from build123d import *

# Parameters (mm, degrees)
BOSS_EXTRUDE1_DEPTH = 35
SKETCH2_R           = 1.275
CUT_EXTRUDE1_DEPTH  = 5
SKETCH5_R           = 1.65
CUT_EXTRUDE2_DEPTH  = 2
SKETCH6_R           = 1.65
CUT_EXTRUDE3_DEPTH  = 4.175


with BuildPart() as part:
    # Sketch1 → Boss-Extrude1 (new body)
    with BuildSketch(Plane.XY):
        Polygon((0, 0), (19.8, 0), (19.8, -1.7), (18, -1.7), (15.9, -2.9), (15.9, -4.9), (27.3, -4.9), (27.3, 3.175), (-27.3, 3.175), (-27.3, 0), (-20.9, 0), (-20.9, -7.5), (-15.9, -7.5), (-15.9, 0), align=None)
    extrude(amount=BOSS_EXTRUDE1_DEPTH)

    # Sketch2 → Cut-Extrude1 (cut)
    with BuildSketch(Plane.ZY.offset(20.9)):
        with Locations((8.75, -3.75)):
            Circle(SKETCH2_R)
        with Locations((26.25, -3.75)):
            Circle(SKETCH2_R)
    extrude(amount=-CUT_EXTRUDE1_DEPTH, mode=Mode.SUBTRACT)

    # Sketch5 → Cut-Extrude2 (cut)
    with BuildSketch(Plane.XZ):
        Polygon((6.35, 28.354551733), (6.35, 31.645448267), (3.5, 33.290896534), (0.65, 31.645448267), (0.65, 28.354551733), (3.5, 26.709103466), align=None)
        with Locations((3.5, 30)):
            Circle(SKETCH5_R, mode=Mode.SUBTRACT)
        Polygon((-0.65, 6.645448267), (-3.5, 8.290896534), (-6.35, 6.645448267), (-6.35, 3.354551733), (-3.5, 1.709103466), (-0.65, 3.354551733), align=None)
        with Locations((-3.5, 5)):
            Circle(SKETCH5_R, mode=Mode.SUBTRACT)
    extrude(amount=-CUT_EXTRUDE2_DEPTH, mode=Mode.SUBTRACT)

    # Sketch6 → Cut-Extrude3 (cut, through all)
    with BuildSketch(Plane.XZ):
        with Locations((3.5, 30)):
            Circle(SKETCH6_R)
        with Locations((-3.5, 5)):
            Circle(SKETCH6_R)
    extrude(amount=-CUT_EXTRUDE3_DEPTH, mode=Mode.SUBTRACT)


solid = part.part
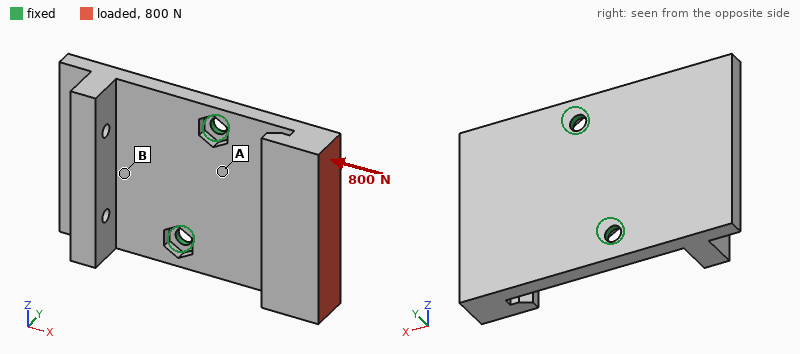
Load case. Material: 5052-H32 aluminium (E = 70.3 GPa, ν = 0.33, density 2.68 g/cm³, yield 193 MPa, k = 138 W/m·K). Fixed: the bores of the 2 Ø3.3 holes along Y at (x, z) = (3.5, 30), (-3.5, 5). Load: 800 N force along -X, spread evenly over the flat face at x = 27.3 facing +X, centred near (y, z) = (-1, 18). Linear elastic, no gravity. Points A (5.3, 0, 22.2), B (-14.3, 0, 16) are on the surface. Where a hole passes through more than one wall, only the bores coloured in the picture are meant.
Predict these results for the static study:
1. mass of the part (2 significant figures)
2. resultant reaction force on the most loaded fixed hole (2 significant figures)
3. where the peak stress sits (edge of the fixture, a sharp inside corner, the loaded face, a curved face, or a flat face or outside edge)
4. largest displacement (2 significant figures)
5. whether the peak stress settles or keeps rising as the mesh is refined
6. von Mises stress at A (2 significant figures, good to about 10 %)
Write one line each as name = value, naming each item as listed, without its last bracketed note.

mass of the part = 24 g
resultant reaction force on the most loaded fixed hole = 400 N
where the peak stress sits = edge of the fixture
largest displacement = 0.25 mm
whether the peak stress settles or keeps rising as the mesh is refined = keeps rising
von Mises stress at A = 43 MPa
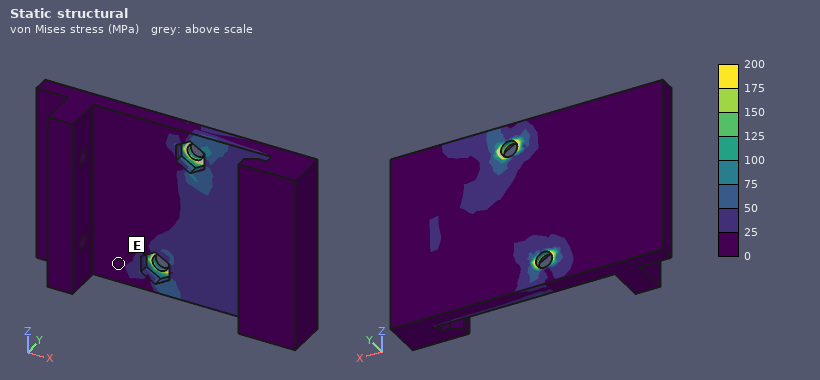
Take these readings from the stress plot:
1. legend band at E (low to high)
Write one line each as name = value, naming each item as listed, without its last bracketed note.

legend band at E = 0 to 25 MPa
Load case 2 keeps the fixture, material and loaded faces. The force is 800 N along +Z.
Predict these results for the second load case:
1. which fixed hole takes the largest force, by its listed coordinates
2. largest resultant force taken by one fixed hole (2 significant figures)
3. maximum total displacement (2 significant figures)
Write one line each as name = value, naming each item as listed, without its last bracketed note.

which fixed hole takes the largest force, by its listed coordinates = (3.5, 30)
largest resultant force taken by one fixed hole = 970 N
maximum total displacement = 88 µm
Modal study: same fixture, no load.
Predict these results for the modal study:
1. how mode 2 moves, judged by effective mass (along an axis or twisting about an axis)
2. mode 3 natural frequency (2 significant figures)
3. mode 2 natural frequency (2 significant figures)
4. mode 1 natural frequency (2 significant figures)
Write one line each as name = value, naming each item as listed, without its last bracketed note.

how mode 2 moves, judged by effective mass = along Y
mode 3 natural frequency = 4800 Hz
mode 2 natural frequency = 2500 Hz
mode 1 natural frequency = 1300 Hz
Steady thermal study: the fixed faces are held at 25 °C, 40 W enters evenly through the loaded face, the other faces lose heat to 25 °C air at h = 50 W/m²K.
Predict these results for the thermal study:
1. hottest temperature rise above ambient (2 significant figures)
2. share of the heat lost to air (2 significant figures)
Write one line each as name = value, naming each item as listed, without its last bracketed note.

hottest temperature rise above ambient = 68 K
share of the heat lost to air = 19 %
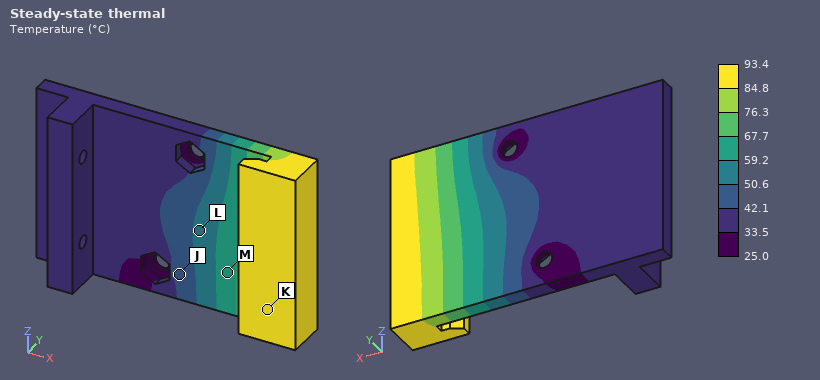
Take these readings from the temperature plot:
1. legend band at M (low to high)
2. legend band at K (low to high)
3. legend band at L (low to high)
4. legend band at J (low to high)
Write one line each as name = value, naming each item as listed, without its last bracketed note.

legend band at M = 59.2 to 67.7 °C
legend band at K = 84.8 to 93.4 °C
legend band at L = 50.6 to 59.2 °C
legend band at J = 42.1 to 50.6 °C
